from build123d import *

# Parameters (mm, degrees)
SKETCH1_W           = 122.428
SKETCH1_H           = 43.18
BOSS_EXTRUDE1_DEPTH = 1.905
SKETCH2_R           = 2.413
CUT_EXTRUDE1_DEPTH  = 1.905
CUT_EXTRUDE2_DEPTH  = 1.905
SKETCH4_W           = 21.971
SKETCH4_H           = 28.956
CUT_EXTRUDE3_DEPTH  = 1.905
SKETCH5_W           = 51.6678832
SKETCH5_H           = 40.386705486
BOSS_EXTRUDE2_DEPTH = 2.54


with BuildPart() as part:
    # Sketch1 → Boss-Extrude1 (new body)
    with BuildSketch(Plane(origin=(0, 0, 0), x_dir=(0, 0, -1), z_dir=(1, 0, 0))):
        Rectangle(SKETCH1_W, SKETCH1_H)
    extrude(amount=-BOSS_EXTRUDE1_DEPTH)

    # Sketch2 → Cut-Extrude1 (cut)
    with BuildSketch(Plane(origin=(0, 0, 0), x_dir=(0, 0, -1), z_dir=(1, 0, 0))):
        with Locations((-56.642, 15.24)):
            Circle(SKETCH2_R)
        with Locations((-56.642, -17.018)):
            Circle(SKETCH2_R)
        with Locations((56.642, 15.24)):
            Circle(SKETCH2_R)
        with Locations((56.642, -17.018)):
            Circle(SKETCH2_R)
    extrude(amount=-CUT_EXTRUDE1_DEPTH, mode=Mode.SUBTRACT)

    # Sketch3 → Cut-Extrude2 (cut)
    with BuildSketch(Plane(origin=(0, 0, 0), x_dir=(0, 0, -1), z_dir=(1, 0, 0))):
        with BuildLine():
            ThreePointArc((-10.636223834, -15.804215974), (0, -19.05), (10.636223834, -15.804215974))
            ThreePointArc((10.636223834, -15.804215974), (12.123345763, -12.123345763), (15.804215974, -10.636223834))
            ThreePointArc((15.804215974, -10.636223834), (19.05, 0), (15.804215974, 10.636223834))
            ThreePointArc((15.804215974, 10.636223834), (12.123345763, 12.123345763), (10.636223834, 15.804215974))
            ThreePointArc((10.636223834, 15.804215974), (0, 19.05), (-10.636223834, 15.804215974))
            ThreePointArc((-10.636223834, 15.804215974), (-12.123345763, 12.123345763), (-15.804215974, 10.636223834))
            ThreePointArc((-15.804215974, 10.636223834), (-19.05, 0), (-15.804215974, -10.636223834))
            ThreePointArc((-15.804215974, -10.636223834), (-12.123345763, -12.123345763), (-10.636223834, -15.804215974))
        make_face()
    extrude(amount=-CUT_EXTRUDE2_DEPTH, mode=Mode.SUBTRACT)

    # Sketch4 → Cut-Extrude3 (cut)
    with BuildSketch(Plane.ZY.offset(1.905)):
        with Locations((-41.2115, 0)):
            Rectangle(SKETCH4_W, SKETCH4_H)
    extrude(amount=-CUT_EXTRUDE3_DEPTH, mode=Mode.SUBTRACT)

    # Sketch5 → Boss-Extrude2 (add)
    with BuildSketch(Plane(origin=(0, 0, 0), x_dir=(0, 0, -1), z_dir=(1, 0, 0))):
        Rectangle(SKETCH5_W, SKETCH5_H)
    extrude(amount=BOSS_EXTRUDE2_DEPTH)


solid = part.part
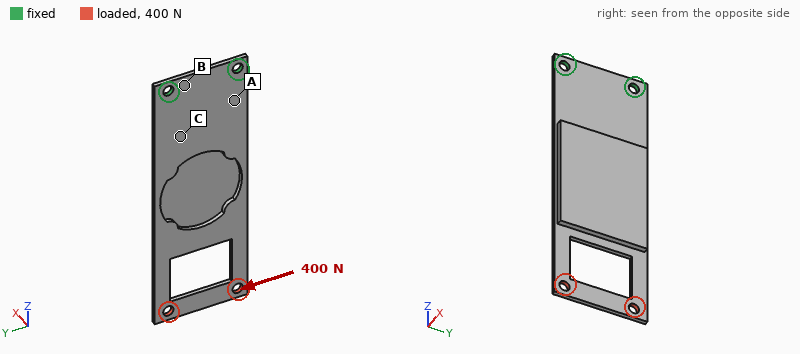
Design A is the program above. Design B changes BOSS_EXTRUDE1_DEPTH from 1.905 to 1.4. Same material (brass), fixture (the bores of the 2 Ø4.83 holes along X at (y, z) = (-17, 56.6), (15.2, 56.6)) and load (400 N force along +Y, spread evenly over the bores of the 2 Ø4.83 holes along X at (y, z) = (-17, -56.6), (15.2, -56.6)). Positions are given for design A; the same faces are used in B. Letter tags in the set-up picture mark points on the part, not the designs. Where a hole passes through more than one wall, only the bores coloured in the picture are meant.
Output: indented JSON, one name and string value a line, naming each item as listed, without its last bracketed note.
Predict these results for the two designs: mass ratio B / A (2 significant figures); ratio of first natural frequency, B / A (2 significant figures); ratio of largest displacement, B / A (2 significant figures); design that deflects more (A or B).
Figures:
{
  "mass ratio B / A": "0.85",
  "ratio of first natural frequency, B / A": "0.71",
  "ratio of largest displacement, B / A": "1.3",
  "design that deflects more": "B"
}
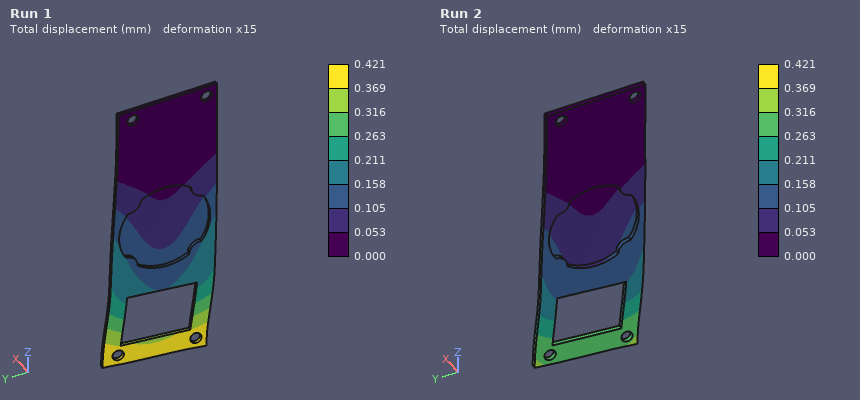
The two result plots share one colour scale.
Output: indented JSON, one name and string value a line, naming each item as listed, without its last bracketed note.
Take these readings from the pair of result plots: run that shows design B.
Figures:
{
  "run that shows design B": "Run 1"
}
